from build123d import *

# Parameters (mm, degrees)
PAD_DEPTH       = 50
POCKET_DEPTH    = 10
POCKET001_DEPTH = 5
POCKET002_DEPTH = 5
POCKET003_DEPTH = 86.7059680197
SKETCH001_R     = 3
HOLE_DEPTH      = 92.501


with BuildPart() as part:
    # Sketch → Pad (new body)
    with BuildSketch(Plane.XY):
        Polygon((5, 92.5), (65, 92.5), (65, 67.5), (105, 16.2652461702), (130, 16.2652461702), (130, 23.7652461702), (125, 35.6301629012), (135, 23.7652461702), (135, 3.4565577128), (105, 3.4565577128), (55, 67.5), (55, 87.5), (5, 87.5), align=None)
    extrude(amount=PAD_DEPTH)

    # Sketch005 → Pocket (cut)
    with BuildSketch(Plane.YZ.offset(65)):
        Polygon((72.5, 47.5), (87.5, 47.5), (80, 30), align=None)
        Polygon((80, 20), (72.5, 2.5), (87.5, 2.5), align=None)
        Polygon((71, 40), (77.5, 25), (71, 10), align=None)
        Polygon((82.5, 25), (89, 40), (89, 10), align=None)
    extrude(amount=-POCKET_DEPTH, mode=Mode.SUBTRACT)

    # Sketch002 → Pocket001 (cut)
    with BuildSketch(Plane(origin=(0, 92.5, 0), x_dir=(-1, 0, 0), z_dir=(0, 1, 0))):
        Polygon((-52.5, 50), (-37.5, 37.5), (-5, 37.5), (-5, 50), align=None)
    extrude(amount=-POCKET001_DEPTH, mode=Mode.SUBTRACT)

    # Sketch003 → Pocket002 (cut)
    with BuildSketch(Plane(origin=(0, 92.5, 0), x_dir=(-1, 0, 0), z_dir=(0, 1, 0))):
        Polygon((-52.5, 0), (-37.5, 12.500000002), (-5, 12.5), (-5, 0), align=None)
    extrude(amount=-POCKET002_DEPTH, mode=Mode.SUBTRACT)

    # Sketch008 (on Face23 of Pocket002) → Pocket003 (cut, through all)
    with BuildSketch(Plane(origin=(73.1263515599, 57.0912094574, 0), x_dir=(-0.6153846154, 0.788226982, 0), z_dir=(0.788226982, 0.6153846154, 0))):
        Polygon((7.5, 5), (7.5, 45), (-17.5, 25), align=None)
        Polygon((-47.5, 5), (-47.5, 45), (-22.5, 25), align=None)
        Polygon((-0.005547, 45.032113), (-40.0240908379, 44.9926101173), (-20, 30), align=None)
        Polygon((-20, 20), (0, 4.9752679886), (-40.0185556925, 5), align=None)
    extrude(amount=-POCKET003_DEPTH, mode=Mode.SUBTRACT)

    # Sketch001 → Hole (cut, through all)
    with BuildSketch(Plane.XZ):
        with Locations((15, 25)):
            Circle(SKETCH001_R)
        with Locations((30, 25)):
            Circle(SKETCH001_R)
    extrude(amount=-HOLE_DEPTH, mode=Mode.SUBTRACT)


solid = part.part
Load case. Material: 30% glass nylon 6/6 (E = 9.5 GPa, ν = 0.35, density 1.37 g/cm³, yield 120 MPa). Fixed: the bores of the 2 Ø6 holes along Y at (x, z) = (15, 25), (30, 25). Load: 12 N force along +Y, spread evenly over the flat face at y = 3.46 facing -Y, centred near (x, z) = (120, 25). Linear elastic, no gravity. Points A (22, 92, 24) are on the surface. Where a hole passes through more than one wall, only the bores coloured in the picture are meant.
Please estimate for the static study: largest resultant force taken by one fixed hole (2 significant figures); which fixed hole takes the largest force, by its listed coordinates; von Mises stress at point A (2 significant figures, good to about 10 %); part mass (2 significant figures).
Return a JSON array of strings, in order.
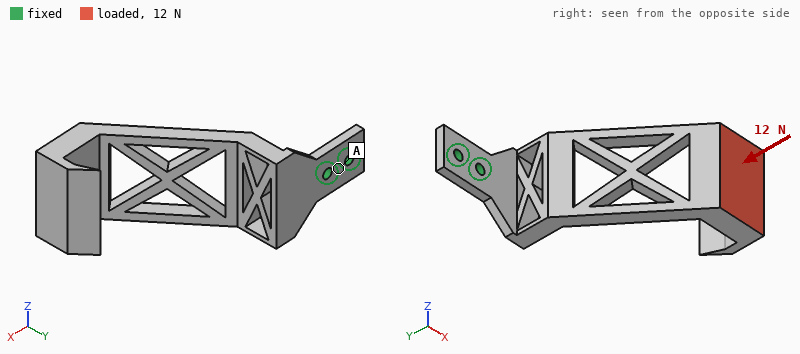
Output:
["29 N", "(30, 25)", "1.3 MPa", "74 g"]
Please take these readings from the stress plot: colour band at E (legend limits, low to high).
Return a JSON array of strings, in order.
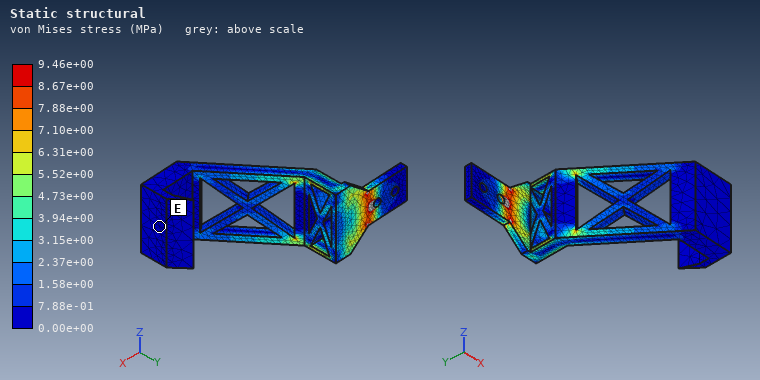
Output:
["0.00e+00 to 7.88e-01 MPa"]
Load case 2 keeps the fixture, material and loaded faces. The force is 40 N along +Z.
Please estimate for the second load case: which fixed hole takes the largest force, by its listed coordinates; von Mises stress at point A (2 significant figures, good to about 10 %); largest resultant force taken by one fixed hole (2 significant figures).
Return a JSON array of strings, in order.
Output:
["(30, 25)", "3.7 MPa", "180 N"]
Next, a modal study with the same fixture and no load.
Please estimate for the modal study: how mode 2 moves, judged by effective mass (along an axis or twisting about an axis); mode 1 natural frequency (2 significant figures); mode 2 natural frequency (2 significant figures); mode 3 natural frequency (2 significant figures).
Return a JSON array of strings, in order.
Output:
["along Z", "60 Hz", "130 Hz", "400 Hz"]
